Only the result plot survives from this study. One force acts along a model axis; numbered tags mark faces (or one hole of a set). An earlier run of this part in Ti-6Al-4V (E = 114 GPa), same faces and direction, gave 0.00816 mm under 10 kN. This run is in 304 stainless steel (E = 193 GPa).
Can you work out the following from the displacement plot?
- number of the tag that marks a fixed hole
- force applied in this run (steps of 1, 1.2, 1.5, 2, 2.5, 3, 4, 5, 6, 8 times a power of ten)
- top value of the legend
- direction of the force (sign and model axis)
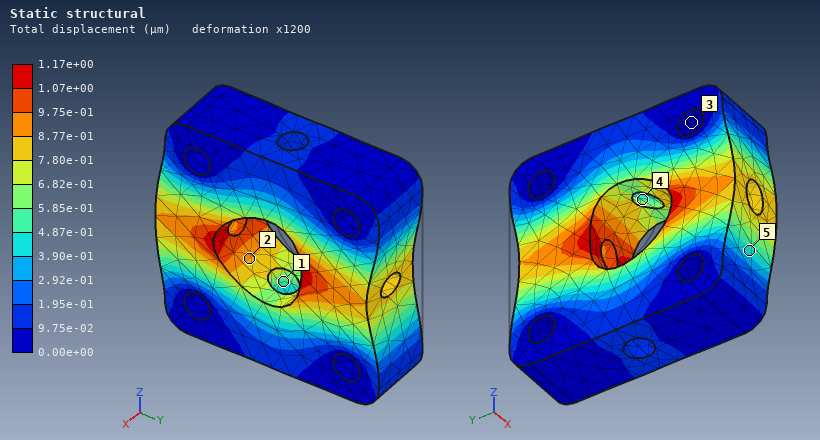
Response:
3
2.5 kN
1.17e+00 µm
-Y
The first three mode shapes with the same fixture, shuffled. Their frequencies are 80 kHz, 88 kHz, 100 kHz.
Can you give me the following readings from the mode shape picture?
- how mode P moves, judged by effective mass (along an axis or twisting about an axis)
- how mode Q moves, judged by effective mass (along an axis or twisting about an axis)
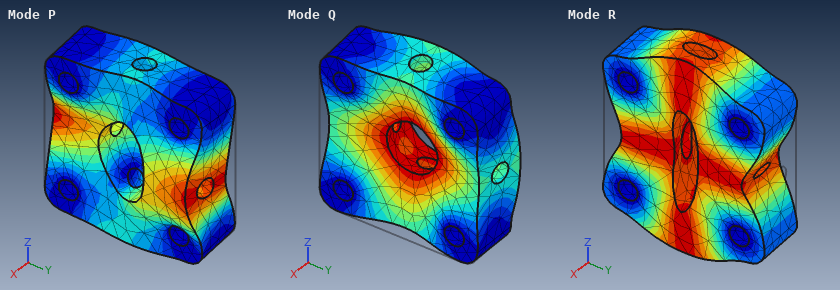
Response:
twisting about Z
along X
